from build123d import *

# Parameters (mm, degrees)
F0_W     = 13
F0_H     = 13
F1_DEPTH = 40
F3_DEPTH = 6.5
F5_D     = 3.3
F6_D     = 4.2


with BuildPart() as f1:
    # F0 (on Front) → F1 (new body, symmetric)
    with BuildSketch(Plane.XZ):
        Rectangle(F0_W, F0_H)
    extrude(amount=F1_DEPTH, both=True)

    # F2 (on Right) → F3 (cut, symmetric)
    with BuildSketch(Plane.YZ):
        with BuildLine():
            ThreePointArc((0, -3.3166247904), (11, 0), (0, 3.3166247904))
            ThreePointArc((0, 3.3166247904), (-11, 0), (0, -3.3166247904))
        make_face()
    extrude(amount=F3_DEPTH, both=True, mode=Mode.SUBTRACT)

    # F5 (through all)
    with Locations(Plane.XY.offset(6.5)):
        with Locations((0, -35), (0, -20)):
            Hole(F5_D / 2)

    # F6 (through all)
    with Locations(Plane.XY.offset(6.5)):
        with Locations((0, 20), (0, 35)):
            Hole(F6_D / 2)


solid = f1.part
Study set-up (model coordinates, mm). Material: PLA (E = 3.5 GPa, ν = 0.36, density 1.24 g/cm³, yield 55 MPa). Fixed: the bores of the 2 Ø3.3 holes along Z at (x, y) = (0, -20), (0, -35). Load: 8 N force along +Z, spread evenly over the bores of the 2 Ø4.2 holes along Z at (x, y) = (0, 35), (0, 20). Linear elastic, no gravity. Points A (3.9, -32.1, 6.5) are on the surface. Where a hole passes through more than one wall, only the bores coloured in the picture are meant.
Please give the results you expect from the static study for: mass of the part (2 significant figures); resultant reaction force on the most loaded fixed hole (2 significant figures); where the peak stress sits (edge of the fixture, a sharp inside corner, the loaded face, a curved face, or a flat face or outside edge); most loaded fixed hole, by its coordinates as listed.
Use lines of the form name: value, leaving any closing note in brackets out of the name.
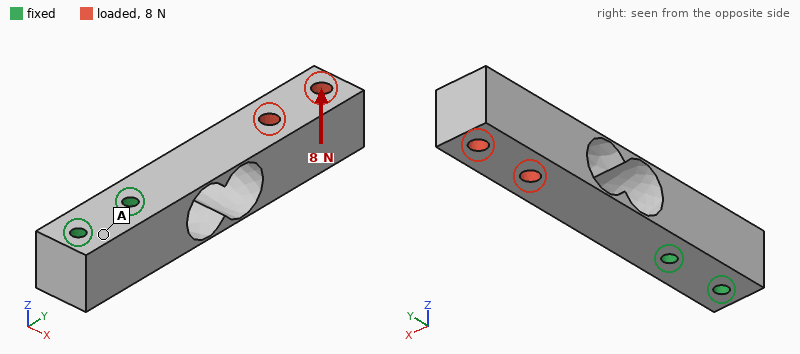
mass of the part: 13 g
resultant reaction force on the most loaded fixed hole: 12 N
where the peak stress sits: a curved face
most loaded fixed hole, by its coordinates as listed: (0, -20)
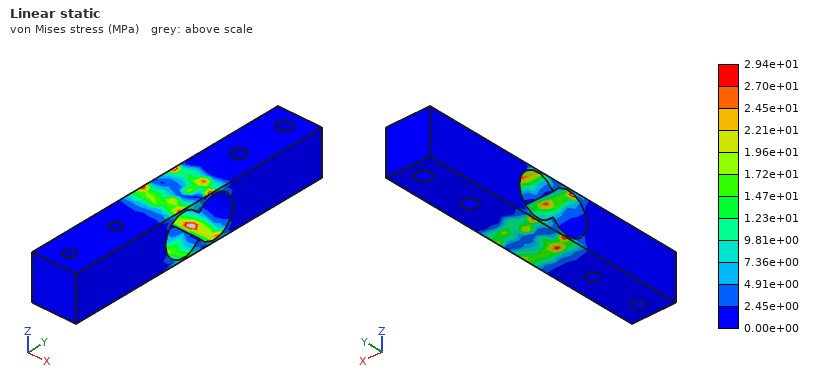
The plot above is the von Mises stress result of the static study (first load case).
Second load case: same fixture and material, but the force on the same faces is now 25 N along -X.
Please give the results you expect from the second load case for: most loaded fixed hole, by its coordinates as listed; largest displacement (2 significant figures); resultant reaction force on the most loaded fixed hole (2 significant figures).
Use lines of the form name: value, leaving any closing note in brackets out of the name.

most loaded fixed hole, by its coordinates as listed: (0, -20)
largest displacement: 0.84 mm
resultant reaction force on the most loaded fixed hole: 74 N
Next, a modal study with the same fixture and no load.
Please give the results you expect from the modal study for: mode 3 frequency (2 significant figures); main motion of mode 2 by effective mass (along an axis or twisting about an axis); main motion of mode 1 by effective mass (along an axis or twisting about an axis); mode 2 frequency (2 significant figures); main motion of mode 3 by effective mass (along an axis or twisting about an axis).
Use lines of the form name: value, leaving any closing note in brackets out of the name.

mode 3 frequency: 1600 Hz
main motion of mode 2 by effective mass: along X
main motion of mode 1 by effective mass: along Z
mode 2 frequency: 440 Hz
main motion of mode 3 by effective mass: twisting about Y
